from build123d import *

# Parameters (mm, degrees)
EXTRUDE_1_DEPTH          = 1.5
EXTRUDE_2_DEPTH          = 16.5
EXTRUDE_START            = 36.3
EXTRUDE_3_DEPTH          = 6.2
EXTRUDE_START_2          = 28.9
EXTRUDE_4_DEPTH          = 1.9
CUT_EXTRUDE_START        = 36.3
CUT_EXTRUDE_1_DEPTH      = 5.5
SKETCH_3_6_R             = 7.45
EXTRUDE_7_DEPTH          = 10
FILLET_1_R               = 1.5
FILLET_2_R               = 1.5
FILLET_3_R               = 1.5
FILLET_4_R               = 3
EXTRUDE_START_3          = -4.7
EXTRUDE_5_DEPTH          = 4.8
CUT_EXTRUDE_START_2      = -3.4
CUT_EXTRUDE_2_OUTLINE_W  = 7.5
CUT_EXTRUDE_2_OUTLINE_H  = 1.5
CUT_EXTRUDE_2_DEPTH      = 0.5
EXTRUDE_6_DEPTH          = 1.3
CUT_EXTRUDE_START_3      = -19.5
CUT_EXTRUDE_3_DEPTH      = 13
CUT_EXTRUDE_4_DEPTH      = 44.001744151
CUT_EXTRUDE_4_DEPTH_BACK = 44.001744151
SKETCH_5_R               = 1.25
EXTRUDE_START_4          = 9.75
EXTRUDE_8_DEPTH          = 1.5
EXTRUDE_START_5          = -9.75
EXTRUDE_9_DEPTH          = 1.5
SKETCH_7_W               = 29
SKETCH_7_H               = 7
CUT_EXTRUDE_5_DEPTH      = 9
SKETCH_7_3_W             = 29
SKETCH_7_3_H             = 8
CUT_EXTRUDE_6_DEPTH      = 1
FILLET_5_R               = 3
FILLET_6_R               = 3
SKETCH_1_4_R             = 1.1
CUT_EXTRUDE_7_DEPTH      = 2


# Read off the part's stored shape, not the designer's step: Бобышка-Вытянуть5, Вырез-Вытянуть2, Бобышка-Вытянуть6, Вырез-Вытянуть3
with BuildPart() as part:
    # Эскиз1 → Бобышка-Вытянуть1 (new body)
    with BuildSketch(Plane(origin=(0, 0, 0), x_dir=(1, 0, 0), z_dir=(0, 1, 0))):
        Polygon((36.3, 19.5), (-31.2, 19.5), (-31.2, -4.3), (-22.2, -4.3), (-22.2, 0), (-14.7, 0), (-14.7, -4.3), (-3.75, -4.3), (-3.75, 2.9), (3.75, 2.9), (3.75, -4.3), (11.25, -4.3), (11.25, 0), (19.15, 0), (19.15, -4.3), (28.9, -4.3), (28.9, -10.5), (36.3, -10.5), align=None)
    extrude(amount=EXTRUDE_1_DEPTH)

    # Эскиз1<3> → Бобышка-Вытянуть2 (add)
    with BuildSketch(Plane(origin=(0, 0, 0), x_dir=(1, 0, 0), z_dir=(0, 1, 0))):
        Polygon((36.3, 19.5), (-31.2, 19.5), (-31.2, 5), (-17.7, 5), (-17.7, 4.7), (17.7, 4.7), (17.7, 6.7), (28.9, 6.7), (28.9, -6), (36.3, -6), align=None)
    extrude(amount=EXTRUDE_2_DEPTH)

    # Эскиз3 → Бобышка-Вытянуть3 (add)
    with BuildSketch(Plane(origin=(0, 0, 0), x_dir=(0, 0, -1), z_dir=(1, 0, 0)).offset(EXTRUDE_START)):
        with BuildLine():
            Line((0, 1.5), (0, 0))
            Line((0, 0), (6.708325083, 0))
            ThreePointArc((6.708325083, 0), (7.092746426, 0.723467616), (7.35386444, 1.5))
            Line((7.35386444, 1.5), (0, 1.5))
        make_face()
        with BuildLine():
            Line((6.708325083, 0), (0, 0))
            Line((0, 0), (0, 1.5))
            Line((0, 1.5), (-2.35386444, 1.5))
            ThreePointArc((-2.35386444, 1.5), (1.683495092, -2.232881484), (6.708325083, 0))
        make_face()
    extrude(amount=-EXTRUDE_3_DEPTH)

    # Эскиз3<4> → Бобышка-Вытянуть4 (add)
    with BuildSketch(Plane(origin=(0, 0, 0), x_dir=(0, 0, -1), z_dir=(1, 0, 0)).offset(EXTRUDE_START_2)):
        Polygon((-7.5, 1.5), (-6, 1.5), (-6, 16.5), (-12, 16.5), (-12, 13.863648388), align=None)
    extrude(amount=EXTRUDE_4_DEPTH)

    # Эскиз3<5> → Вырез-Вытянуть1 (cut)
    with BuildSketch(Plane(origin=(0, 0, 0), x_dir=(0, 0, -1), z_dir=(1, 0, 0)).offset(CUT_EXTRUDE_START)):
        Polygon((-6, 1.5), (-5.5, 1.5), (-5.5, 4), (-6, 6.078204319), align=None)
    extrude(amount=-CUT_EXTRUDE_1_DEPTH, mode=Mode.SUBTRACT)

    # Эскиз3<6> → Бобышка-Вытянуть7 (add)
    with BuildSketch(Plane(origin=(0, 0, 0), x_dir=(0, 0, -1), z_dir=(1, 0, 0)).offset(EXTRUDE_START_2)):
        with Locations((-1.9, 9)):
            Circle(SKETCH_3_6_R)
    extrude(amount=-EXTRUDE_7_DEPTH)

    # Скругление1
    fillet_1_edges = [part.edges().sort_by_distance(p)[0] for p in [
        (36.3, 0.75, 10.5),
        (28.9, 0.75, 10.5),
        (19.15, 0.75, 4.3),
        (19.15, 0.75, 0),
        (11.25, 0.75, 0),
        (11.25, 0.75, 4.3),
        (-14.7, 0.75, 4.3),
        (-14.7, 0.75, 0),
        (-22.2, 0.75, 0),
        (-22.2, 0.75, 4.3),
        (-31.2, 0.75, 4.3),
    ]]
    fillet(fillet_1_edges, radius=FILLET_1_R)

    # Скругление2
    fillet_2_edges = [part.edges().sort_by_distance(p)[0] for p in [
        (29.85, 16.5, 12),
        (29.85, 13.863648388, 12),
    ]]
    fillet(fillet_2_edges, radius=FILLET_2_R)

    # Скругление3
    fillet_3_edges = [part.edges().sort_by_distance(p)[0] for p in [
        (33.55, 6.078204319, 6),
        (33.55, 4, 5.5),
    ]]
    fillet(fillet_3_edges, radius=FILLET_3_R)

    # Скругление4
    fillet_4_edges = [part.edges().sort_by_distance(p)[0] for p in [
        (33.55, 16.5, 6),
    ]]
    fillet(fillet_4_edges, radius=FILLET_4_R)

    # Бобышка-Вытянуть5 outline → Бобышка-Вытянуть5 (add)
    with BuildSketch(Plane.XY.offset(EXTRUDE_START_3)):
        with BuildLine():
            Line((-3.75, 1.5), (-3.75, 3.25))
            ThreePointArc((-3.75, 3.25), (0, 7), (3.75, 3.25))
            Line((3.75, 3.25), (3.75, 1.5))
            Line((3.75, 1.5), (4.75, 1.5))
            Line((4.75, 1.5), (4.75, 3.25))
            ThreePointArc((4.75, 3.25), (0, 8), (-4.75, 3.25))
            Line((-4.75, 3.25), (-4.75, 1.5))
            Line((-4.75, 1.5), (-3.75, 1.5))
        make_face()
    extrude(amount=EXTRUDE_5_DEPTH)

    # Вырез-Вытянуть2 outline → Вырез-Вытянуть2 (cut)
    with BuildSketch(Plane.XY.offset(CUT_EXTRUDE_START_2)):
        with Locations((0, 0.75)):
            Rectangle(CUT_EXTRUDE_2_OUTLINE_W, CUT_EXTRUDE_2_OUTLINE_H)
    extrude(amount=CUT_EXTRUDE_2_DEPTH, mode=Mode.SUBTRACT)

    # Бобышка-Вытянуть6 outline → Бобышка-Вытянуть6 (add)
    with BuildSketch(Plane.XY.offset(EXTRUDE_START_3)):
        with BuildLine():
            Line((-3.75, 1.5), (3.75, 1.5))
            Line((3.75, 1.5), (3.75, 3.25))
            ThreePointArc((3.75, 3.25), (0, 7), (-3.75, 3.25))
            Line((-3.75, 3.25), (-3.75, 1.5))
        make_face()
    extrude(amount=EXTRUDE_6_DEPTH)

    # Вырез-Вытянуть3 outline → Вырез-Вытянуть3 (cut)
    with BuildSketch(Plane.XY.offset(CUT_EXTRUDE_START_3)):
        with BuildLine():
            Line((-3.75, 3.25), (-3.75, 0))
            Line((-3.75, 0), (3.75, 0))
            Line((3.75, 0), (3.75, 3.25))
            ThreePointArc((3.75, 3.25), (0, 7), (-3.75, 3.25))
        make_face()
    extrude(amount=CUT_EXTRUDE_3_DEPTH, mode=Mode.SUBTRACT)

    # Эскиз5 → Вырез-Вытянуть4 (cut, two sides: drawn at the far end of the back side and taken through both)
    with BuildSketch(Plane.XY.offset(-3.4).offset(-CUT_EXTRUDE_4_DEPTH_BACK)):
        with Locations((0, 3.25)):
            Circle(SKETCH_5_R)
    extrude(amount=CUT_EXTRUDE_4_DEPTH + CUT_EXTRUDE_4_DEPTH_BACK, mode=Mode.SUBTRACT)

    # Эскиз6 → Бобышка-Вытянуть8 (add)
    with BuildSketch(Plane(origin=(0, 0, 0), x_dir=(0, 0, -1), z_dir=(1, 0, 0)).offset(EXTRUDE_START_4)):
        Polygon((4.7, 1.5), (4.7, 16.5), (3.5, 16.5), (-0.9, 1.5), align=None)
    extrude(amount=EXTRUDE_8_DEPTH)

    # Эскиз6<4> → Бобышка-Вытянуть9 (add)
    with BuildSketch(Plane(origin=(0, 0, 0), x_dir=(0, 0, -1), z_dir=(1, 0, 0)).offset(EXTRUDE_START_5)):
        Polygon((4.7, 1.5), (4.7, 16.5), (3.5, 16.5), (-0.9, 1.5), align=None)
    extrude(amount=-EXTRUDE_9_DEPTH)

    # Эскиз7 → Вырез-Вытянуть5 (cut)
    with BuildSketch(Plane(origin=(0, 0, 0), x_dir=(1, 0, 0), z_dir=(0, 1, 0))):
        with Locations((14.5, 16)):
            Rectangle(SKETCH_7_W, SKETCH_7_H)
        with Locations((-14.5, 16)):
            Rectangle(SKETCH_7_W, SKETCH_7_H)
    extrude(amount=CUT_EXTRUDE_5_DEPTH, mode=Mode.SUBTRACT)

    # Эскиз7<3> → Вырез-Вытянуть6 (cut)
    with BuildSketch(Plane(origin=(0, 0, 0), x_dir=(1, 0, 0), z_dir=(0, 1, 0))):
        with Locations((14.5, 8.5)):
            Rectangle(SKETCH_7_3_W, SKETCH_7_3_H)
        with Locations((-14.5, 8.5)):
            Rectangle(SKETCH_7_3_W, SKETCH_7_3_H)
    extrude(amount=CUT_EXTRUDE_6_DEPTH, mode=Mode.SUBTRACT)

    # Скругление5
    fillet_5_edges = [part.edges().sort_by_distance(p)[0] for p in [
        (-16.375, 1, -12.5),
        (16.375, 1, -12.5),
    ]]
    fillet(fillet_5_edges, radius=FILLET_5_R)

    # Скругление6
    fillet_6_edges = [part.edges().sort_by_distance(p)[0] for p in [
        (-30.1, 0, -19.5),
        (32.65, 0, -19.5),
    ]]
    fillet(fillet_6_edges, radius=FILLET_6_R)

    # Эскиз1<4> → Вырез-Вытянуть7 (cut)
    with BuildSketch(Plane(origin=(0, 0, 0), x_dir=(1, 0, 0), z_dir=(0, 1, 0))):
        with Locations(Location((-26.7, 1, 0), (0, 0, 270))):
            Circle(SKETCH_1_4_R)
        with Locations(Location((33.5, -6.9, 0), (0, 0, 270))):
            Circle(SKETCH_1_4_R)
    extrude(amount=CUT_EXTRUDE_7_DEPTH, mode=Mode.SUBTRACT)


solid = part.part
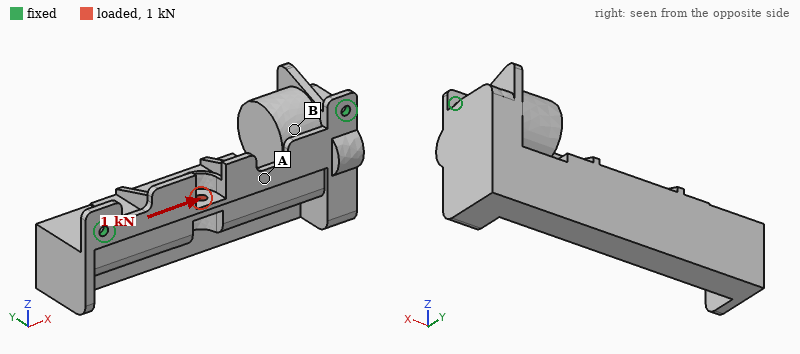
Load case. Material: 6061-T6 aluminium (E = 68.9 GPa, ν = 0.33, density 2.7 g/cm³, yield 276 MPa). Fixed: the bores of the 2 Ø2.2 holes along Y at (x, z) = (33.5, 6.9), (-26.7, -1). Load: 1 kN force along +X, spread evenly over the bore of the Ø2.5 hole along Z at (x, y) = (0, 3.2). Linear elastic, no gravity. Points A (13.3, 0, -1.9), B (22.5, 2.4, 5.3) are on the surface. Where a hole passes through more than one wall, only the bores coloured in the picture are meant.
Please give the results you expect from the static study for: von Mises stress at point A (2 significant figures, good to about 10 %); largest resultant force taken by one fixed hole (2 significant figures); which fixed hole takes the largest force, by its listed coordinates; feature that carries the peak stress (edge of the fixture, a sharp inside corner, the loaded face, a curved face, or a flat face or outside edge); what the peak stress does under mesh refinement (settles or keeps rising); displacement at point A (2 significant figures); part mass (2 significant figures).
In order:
23 MPa
670 N
(-26.7, -1)
edge of the fixture
keeps rising
20 µm
43 g
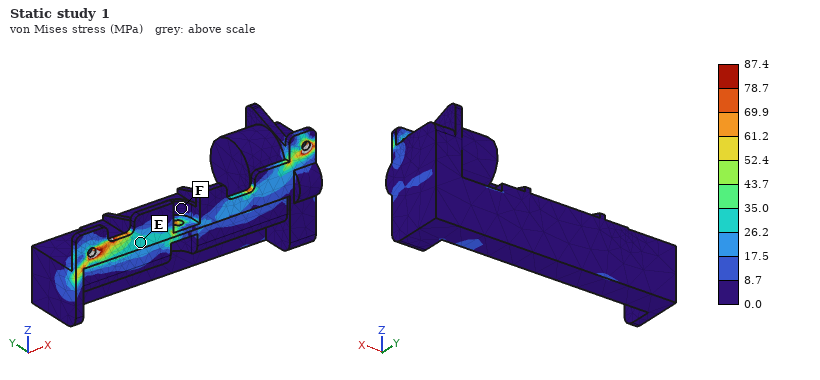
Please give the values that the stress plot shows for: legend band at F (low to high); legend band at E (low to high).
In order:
0.0 to 8.7 MPa
26.2 to 35.0 MPa
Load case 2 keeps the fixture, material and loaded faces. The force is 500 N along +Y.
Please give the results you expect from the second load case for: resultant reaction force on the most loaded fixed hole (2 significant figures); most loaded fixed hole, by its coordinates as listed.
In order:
300 N
(-26.7, -1)
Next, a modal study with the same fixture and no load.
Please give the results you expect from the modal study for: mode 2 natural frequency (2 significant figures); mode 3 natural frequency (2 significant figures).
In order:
4400 Hz
6000 Hz
